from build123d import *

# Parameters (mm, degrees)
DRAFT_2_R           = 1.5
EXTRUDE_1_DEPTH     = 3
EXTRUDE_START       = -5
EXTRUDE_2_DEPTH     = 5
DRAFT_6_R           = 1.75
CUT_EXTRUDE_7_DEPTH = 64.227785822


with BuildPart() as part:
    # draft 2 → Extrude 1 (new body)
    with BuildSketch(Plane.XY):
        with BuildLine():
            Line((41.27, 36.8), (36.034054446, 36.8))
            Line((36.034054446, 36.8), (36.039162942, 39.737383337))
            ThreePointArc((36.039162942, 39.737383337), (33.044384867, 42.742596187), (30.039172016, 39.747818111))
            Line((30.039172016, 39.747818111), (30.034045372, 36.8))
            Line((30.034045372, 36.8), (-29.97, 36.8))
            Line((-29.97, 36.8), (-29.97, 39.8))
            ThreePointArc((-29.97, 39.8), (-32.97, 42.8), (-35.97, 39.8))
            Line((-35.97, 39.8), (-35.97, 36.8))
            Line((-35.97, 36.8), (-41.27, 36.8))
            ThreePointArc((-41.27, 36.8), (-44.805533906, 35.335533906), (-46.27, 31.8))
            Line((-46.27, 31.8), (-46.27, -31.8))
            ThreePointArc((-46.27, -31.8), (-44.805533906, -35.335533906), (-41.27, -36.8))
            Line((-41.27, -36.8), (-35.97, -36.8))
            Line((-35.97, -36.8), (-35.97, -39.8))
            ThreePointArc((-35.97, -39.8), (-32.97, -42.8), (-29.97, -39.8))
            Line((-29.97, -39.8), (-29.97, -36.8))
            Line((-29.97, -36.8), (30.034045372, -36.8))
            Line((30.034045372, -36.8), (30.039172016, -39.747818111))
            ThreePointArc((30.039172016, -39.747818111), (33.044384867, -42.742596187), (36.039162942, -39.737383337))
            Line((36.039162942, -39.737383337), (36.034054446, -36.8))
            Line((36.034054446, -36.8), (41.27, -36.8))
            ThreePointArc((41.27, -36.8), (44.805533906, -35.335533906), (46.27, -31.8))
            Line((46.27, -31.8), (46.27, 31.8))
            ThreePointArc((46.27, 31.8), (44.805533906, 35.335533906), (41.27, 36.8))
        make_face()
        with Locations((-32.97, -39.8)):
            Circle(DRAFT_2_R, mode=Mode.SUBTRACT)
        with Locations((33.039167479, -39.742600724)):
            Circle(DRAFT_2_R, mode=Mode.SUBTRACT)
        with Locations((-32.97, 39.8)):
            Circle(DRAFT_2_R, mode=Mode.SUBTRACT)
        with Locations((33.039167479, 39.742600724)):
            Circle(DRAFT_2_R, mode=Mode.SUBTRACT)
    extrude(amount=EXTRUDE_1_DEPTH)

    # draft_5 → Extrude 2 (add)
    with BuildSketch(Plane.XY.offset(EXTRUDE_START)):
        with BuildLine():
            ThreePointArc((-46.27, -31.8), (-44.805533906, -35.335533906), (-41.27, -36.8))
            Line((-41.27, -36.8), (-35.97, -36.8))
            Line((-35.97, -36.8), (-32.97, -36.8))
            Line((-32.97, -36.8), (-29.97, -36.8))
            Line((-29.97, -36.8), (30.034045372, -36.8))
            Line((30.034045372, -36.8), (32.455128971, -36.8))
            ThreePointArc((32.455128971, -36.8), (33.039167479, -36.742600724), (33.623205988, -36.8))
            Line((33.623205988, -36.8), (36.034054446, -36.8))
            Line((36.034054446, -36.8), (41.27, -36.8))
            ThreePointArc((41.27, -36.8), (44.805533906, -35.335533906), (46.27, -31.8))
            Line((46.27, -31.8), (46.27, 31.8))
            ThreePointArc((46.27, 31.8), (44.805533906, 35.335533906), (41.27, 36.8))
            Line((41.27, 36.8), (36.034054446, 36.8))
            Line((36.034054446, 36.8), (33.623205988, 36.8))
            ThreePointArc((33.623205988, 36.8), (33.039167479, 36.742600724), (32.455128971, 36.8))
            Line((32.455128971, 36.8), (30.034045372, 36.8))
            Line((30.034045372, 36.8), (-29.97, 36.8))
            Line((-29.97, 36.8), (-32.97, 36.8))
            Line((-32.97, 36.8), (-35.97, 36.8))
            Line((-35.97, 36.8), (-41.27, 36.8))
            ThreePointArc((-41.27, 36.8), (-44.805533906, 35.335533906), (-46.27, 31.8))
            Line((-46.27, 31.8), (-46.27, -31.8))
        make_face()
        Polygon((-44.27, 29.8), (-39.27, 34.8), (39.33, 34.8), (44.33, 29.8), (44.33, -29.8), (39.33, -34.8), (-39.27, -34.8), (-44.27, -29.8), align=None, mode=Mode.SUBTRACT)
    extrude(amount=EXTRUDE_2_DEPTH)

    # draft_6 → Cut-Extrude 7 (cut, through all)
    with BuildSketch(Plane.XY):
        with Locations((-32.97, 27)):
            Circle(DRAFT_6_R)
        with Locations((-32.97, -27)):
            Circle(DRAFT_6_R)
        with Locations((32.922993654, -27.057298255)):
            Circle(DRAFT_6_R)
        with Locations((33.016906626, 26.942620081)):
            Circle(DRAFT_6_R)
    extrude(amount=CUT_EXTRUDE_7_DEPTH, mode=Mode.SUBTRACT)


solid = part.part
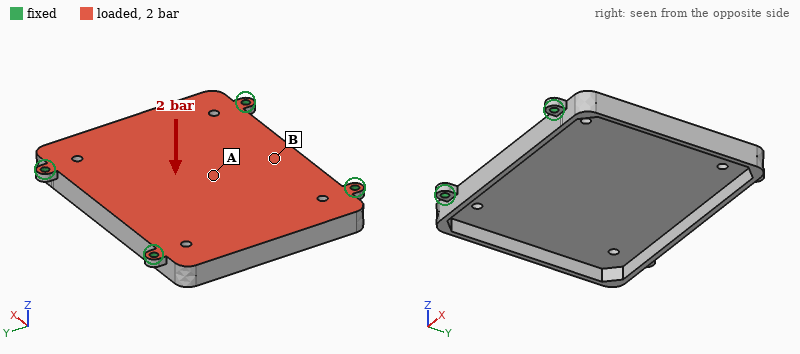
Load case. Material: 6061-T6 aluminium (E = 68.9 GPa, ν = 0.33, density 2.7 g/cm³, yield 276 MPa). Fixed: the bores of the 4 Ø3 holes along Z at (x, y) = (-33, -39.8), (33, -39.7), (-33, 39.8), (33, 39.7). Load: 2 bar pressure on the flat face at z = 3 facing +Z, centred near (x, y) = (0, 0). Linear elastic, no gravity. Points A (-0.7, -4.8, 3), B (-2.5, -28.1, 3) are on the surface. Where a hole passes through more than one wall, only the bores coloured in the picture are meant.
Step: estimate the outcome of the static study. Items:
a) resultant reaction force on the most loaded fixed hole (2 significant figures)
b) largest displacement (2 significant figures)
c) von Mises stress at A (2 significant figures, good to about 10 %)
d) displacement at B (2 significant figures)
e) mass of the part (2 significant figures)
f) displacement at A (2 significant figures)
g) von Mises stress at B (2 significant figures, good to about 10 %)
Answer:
360 N
0.24 mm
43 MPa
0.12 mm
65 g
0.24 mm
22 MPa
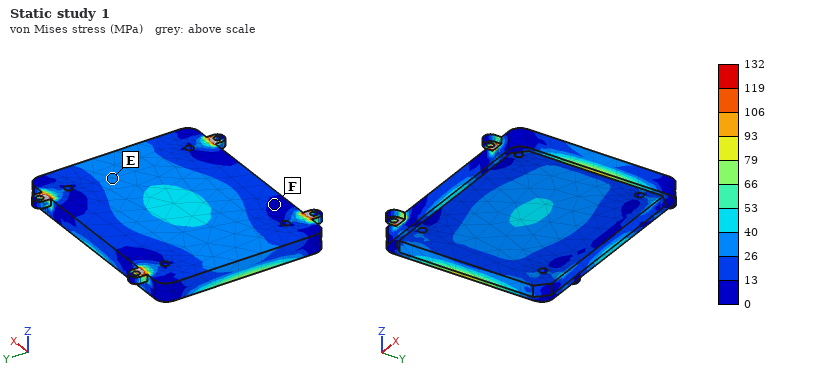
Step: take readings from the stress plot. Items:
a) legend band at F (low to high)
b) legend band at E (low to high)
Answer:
0 to 13 MPa
26 to 40 MPa
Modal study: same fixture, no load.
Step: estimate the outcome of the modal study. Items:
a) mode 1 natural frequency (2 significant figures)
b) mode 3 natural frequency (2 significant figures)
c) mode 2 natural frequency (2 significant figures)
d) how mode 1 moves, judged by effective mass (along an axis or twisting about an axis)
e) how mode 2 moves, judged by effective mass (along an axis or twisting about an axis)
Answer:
1900 Hz
3200 Hz
2800 Hz
along Z
twisting about Y
